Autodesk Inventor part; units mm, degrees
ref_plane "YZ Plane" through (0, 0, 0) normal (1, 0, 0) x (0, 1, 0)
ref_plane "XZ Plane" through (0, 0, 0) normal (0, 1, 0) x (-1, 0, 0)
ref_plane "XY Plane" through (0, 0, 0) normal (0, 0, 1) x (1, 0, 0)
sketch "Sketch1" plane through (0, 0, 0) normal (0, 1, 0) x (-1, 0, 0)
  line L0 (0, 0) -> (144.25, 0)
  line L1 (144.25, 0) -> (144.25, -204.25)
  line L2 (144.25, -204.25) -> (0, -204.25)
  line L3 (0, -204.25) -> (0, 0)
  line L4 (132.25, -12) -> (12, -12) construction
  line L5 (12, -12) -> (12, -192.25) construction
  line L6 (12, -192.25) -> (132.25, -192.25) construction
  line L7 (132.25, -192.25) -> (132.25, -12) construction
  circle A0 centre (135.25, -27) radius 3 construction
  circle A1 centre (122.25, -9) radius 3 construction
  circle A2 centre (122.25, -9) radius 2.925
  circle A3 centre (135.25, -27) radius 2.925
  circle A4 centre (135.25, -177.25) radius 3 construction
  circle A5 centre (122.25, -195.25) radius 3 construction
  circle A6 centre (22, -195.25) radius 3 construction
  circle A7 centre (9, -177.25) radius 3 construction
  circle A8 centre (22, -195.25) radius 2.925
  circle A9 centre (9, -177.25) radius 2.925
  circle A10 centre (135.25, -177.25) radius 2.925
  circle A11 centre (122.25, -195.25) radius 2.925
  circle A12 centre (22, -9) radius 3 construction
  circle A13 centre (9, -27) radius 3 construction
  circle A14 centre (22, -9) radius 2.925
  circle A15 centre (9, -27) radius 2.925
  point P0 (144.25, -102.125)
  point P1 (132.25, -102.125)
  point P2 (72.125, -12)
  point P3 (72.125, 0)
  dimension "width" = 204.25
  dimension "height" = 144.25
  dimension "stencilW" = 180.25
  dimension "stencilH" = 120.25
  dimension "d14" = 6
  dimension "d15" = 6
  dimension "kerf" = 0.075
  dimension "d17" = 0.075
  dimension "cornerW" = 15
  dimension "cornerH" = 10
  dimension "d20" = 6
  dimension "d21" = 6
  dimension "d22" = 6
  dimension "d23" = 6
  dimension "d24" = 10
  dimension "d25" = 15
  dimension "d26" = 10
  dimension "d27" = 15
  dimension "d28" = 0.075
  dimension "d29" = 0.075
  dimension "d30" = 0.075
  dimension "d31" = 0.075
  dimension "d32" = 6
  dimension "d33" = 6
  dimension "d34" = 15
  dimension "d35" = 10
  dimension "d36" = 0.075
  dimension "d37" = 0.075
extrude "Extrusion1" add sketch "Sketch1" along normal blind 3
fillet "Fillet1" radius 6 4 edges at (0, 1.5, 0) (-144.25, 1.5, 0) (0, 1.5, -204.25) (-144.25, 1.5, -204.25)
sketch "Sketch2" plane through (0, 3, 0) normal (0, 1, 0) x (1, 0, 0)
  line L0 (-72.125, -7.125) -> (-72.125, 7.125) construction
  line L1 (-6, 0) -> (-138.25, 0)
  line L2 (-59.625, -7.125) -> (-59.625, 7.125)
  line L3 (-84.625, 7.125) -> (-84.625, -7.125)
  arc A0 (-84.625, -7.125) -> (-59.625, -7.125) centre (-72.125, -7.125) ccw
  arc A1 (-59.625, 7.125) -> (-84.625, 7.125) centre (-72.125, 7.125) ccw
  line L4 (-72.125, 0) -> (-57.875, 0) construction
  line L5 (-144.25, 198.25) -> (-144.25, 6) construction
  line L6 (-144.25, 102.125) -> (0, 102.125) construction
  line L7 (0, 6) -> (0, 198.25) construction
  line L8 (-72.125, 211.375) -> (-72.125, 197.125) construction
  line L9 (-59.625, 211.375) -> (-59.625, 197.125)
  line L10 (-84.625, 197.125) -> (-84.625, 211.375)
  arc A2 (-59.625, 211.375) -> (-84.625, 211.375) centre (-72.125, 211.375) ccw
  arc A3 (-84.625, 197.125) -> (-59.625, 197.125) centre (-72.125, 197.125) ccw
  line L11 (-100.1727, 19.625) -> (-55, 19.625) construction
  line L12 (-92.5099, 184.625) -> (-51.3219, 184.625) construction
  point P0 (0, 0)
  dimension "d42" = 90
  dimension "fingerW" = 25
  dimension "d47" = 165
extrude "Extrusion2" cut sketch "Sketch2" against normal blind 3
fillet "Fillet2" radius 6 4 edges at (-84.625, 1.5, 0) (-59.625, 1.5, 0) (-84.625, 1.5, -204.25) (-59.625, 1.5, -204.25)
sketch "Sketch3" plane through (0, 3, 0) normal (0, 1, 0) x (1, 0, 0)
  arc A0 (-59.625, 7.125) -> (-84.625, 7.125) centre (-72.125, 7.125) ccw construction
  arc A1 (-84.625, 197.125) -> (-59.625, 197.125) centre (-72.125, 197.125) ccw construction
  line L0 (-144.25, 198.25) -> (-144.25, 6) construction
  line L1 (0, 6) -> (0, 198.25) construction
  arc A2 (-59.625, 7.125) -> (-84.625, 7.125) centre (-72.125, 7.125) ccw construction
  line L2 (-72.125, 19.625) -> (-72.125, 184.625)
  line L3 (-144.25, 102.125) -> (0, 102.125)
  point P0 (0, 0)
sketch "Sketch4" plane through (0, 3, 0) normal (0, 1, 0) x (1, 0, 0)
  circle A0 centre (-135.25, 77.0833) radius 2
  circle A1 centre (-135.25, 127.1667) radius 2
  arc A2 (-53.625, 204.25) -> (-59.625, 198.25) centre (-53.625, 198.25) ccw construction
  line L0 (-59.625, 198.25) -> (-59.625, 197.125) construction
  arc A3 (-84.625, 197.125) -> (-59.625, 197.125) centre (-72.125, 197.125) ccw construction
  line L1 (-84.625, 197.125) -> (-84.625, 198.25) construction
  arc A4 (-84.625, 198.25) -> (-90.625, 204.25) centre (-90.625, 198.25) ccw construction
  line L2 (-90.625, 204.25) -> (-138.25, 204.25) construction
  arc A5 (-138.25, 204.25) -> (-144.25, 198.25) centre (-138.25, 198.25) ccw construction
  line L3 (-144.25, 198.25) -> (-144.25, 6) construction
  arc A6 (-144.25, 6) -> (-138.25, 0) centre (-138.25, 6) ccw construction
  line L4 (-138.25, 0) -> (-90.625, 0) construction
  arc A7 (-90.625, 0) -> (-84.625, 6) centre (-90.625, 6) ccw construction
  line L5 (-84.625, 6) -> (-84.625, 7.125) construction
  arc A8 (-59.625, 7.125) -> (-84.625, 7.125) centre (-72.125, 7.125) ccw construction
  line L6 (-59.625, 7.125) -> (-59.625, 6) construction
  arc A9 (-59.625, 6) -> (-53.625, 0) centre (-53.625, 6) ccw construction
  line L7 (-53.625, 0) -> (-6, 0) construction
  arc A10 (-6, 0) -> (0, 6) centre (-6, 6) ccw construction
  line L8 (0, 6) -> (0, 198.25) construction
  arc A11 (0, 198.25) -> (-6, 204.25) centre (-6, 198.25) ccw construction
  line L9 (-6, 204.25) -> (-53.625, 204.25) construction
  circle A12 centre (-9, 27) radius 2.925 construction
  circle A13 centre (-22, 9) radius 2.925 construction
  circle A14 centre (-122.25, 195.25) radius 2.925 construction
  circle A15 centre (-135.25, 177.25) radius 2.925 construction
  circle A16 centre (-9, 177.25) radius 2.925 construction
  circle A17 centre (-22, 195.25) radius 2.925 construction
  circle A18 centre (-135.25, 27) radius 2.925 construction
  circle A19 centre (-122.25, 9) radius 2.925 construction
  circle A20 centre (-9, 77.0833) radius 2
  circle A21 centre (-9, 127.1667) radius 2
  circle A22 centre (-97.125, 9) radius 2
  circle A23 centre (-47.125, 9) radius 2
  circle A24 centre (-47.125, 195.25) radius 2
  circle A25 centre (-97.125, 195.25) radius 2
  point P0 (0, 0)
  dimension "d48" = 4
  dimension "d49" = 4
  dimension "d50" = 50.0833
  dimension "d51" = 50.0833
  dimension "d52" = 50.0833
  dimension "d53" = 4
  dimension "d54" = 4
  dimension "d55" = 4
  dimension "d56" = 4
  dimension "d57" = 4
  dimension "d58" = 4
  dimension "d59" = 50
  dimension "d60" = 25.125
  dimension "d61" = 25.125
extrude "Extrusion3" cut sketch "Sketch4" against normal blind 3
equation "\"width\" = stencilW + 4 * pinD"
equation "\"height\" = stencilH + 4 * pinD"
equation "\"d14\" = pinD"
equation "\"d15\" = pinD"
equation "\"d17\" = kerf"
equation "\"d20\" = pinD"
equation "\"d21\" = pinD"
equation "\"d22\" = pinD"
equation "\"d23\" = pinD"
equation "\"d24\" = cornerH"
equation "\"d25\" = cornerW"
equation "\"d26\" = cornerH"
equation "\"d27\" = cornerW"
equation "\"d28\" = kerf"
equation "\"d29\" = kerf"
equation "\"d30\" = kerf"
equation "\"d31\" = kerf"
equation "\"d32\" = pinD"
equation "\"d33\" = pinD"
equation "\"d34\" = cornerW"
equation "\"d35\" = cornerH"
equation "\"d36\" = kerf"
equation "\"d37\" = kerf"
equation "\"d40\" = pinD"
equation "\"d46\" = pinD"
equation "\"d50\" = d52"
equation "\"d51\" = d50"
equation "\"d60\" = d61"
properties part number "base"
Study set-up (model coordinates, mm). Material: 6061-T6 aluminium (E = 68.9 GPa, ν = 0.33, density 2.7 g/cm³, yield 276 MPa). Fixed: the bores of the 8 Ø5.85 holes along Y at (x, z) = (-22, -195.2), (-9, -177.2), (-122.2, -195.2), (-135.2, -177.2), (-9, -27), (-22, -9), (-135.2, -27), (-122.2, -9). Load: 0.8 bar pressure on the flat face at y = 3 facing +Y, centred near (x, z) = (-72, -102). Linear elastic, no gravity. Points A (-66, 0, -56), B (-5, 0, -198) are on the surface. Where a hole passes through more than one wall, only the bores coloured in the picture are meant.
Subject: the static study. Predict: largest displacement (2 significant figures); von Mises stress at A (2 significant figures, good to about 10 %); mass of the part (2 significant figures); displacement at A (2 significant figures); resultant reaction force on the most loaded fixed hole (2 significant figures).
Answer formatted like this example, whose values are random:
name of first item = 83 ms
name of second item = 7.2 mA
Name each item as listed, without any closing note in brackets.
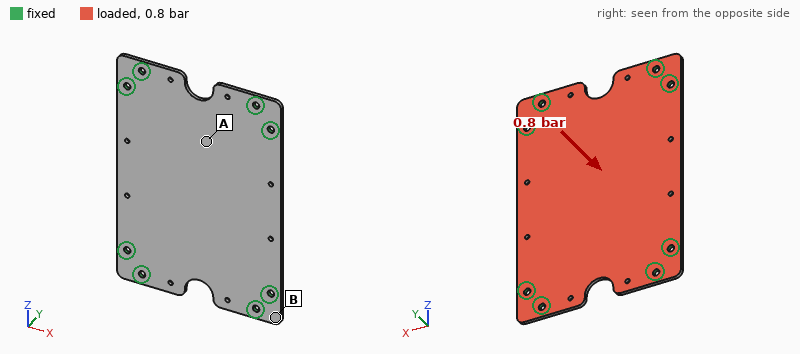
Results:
largest displacement = 1.2 mm
von Mises stress at A = 37 MPa
mass of the part = 230 g
displacement at A = 0.82 mm
resultant reaction force on the most loaded fixed hole = 470 N
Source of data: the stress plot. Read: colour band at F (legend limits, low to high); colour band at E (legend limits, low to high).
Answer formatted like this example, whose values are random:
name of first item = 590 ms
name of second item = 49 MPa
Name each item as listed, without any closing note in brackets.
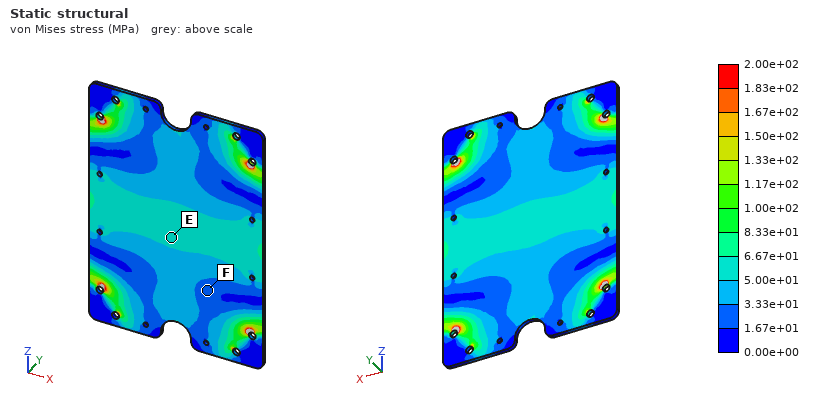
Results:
colour band at F = 1.67e+01 to 3.33e+01 MPa
colour band at E = 5.00e+01 to 6.67e+01 MPa
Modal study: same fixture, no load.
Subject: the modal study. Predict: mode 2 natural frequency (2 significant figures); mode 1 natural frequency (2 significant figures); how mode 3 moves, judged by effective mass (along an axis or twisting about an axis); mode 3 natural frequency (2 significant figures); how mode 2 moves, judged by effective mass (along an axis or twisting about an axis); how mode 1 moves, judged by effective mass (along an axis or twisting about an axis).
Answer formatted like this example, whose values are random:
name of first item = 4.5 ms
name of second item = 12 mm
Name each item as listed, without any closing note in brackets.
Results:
mode 2 natural frequency = 840 Hz
mode 1 natural frequency = 540 Hz
how mode 3 moves, judged by effective mass = twisting about X
mode 3 natural frequency = 1200 Hz
how mode 2 moves, judged by effective mass = twisting about Z
how mode 1 moves, judged by effective mass = along Y
